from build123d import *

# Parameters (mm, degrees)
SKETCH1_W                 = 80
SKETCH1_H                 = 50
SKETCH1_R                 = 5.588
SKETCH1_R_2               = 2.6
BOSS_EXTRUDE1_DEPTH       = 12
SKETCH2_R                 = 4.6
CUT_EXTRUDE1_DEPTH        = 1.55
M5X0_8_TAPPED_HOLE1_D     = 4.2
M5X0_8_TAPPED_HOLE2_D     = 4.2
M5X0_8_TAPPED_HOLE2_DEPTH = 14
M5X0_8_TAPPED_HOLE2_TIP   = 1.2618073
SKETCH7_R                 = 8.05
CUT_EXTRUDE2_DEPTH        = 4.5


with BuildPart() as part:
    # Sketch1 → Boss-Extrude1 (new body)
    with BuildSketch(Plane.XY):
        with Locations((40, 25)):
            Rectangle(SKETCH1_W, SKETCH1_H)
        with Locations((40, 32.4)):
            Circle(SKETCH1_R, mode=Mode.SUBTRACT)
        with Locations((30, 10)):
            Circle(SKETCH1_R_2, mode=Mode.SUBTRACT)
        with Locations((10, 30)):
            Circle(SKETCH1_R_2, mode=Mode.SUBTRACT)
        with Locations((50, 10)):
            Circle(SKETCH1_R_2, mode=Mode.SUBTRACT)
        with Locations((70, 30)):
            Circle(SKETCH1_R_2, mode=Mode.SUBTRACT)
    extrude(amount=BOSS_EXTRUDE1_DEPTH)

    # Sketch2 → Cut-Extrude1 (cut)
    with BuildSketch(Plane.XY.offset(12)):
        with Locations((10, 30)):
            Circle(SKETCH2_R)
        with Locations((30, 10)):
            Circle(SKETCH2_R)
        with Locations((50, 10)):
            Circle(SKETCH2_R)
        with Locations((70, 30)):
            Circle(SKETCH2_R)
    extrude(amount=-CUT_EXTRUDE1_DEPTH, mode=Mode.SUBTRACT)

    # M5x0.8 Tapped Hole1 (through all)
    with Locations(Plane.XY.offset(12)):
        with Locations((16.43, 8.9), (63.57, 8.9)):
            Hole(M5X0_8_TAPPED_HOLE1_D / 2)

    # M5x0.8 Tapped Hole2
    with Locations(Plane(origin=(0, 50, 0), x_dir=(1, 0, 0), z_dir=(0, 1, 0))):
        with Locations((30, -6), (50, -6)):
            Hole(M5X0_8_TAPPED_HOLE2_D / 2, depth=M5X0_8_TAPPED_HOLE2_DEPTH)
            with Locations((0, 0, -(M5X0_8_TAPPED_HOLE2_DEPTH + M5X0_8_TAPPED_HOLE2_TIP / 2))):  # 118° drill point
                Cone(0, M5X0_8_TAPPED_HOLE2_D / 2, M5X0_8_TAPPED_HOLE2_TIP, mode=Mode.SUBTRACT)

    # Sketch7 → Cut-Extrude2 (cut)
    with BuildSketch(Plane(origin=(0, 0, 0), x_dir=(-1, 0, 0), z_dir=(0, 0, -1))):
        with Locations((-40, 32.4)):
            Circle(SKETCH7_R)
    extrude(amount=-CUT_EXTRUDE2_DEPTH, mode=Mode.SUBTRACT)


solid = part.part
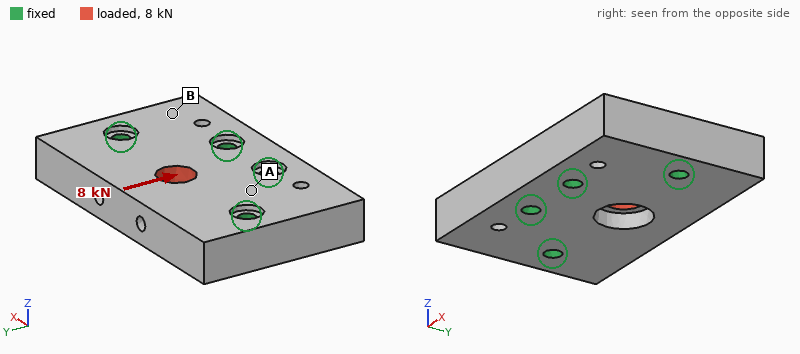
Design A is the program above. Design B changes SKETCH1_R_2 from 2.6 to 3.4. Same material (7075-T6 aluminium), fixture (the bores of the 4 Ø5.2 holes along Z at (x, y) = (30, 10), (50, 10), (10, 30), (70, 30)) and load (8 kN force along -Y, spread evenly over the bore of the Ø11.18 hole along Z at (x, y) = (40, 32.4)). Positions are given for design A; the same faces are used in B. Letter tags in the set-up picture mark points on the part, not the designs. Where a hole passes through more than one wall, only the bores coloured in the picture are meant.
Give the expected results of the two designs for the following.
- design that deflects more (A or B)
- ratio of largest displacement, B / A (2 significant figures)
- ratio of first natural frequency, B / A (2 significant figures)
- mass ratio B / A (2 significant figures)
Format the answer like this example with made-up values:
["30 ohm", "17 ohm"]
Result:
["A", "0.92", "1.1", "0.99"]
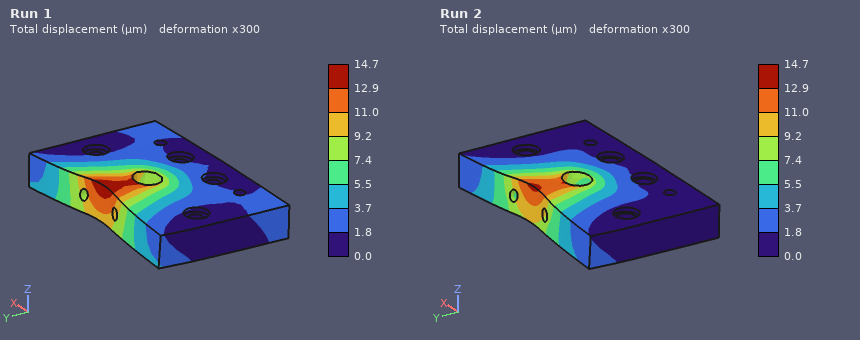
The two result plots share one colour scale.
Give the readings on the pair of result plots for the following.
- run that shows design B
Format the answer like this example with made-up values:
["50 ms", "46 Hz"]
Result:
["Run 2"]
